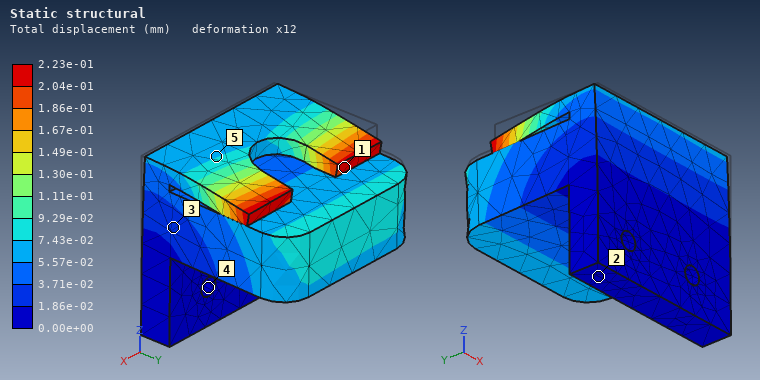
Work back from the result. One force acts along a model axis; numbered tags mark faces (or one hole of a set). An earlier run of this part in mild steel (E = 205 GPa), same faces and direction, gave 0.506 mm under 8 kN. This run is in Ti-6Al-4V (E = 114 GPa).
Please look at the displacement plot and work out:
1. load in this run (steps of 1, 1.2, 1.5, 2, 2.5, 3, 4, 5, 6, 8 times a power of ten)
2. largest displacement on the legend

2 kN
2.23e-01 mm
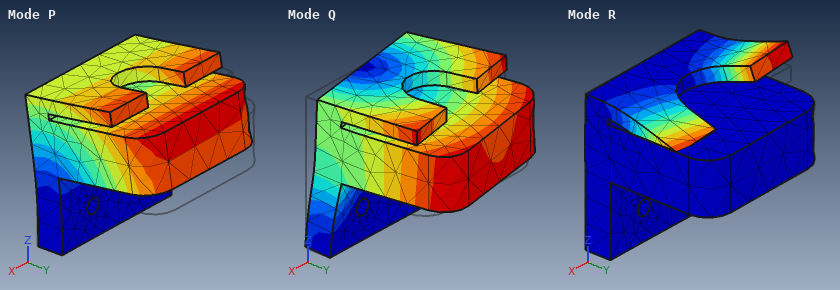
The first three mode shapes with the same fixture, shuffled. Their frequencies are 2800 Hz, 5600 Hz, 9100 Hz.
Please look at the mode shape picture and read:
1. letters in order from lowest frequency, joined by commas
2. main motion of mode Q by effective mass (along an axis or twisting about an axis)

P, Q, R
along X
